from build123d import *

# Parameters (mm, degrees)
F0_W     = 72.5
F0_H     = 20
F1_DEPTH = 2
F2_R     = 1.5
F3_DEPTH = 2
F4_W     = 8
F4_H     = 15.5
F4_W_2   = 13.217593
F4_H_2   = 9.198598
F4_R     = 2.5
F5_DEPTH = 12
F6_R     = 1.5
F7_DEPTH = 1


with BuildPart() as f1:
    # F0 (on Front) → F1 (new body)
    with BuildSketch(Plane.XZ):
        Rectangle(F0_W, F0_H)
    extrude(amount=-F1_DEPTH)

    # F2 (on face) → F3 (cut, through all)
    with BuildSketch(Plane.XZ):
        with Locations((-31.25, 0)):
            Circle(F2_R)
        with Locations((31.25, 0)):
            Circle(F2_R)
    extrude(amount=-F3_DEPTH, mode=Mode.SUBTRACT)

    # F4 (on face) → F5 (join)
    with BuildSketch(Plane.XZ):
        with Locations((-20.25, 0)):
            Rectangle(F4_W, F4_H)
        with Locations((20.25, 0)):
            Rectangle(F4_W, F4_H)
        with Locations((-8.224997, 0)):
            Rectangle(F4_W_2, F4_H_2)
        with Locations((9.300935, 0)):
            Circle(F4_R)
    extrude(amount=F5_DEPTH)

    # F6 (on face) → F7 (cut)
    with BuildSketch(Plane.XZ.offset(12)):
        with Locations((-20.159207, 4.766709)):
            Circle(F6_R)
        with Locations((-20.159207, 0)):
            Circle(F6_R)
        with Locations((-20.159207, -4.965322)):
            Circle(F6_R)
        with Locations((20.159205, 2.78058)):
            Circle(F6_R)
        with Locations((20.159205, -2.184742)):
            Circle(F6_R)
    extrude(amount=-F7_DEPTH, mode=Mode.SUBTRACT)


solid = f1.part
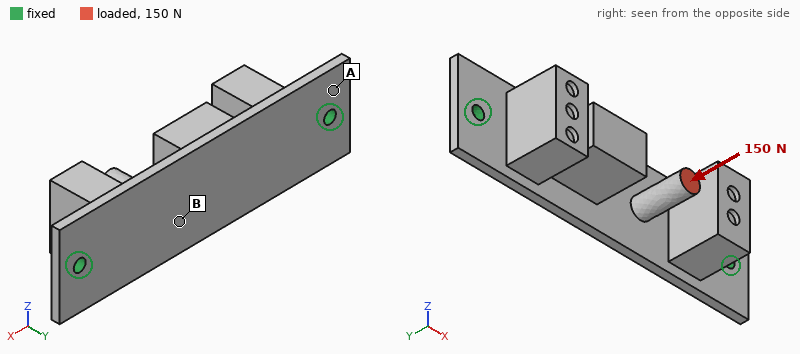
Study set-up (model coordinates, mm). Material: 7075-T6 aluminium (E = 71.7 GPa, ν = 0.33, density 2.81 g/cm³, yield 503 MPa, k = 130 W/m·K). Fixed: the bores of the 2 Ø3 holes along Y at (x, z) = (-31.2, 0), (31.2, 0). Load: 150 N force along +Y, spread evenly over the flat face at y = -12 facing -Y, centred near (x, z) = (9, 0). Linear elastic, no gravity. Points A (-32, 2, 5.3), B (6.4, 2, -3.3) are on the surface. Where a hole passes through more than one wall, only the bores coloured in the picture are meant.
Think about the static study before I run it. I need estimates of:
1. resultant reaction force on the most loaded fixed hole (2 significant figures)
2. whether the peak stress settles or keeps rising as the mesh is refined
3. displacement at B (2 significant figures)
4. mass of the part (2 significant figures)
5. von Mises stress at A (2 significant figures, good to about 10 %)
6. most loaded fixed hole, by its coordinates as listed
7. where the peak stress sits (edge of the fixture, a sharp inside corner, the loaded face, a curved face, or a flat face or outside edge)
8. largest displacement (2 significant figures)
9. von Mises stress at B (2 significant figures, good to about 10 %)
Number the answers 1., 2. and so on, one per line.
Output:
1. 110 N
2. keeps rising
3. 0.14 mm
4. 21 g
5. 20 MPa
6. (31.2, 0)
7. edge of the fixture
8. 0.15 mm
9. 61 MPa
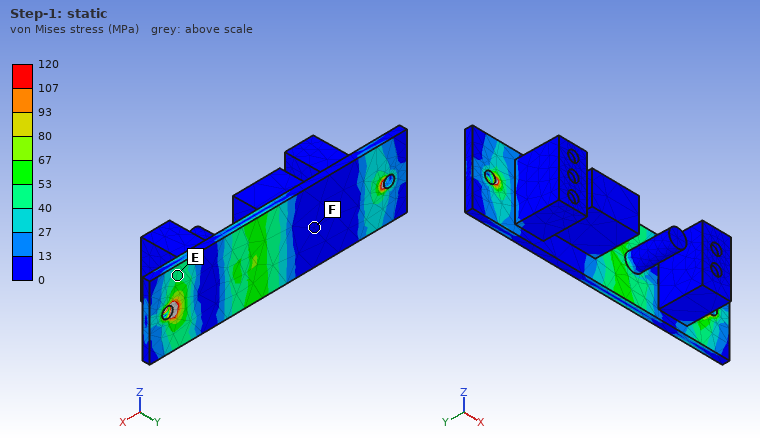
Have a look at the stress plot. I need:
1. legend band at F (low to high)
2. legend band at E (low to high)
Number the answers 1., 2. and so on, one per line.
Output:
1. 0 to 13 MPa
2. 40 to 53 MPa
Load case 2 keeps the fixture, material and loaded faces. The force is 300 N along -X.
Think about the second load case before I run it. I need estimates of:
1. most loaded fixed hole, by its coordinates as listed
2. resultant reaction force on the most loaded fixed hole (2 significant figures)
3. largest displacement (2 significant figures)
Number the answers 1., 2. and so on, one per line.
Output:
1. (31.2, 0)
2. 200 N
3. 0.33 mm
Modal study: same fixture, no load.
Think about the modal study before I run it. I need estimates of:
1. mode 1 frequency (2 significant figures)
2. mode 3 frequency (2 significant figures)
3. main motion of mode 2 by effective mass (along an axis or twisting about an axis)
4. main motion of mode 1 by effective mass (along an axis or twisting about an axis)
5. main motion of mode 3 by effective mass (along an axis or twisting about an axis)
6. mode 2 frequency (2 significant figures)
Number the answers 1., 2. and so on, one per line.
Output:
1. 1700 Hz
2. 4400 Hz
3. along Z
4. along Y
5. twisting about Z
6. 3000 Hz
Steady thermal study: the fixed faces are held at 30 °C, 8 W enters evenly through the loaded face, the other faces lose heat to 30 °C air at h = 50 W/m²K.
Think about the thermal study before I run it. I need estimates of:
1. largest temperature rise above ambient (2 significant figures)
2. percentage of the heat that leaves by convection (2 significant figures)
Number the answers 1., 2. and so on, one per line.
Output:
1. 57 K
2. 26 %
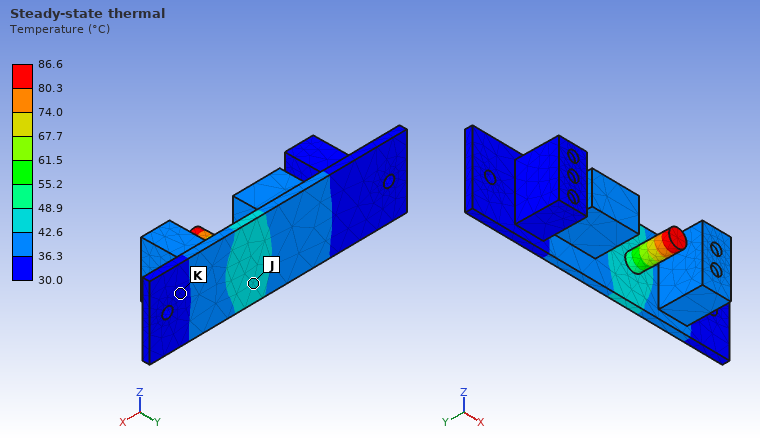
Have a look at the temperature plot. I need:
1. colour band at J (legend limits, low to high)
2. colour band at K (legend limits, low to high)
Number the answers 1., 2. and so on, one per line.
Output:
1. 42.6 to 48.9 °C
2. 30.0 to 36.3 °C
